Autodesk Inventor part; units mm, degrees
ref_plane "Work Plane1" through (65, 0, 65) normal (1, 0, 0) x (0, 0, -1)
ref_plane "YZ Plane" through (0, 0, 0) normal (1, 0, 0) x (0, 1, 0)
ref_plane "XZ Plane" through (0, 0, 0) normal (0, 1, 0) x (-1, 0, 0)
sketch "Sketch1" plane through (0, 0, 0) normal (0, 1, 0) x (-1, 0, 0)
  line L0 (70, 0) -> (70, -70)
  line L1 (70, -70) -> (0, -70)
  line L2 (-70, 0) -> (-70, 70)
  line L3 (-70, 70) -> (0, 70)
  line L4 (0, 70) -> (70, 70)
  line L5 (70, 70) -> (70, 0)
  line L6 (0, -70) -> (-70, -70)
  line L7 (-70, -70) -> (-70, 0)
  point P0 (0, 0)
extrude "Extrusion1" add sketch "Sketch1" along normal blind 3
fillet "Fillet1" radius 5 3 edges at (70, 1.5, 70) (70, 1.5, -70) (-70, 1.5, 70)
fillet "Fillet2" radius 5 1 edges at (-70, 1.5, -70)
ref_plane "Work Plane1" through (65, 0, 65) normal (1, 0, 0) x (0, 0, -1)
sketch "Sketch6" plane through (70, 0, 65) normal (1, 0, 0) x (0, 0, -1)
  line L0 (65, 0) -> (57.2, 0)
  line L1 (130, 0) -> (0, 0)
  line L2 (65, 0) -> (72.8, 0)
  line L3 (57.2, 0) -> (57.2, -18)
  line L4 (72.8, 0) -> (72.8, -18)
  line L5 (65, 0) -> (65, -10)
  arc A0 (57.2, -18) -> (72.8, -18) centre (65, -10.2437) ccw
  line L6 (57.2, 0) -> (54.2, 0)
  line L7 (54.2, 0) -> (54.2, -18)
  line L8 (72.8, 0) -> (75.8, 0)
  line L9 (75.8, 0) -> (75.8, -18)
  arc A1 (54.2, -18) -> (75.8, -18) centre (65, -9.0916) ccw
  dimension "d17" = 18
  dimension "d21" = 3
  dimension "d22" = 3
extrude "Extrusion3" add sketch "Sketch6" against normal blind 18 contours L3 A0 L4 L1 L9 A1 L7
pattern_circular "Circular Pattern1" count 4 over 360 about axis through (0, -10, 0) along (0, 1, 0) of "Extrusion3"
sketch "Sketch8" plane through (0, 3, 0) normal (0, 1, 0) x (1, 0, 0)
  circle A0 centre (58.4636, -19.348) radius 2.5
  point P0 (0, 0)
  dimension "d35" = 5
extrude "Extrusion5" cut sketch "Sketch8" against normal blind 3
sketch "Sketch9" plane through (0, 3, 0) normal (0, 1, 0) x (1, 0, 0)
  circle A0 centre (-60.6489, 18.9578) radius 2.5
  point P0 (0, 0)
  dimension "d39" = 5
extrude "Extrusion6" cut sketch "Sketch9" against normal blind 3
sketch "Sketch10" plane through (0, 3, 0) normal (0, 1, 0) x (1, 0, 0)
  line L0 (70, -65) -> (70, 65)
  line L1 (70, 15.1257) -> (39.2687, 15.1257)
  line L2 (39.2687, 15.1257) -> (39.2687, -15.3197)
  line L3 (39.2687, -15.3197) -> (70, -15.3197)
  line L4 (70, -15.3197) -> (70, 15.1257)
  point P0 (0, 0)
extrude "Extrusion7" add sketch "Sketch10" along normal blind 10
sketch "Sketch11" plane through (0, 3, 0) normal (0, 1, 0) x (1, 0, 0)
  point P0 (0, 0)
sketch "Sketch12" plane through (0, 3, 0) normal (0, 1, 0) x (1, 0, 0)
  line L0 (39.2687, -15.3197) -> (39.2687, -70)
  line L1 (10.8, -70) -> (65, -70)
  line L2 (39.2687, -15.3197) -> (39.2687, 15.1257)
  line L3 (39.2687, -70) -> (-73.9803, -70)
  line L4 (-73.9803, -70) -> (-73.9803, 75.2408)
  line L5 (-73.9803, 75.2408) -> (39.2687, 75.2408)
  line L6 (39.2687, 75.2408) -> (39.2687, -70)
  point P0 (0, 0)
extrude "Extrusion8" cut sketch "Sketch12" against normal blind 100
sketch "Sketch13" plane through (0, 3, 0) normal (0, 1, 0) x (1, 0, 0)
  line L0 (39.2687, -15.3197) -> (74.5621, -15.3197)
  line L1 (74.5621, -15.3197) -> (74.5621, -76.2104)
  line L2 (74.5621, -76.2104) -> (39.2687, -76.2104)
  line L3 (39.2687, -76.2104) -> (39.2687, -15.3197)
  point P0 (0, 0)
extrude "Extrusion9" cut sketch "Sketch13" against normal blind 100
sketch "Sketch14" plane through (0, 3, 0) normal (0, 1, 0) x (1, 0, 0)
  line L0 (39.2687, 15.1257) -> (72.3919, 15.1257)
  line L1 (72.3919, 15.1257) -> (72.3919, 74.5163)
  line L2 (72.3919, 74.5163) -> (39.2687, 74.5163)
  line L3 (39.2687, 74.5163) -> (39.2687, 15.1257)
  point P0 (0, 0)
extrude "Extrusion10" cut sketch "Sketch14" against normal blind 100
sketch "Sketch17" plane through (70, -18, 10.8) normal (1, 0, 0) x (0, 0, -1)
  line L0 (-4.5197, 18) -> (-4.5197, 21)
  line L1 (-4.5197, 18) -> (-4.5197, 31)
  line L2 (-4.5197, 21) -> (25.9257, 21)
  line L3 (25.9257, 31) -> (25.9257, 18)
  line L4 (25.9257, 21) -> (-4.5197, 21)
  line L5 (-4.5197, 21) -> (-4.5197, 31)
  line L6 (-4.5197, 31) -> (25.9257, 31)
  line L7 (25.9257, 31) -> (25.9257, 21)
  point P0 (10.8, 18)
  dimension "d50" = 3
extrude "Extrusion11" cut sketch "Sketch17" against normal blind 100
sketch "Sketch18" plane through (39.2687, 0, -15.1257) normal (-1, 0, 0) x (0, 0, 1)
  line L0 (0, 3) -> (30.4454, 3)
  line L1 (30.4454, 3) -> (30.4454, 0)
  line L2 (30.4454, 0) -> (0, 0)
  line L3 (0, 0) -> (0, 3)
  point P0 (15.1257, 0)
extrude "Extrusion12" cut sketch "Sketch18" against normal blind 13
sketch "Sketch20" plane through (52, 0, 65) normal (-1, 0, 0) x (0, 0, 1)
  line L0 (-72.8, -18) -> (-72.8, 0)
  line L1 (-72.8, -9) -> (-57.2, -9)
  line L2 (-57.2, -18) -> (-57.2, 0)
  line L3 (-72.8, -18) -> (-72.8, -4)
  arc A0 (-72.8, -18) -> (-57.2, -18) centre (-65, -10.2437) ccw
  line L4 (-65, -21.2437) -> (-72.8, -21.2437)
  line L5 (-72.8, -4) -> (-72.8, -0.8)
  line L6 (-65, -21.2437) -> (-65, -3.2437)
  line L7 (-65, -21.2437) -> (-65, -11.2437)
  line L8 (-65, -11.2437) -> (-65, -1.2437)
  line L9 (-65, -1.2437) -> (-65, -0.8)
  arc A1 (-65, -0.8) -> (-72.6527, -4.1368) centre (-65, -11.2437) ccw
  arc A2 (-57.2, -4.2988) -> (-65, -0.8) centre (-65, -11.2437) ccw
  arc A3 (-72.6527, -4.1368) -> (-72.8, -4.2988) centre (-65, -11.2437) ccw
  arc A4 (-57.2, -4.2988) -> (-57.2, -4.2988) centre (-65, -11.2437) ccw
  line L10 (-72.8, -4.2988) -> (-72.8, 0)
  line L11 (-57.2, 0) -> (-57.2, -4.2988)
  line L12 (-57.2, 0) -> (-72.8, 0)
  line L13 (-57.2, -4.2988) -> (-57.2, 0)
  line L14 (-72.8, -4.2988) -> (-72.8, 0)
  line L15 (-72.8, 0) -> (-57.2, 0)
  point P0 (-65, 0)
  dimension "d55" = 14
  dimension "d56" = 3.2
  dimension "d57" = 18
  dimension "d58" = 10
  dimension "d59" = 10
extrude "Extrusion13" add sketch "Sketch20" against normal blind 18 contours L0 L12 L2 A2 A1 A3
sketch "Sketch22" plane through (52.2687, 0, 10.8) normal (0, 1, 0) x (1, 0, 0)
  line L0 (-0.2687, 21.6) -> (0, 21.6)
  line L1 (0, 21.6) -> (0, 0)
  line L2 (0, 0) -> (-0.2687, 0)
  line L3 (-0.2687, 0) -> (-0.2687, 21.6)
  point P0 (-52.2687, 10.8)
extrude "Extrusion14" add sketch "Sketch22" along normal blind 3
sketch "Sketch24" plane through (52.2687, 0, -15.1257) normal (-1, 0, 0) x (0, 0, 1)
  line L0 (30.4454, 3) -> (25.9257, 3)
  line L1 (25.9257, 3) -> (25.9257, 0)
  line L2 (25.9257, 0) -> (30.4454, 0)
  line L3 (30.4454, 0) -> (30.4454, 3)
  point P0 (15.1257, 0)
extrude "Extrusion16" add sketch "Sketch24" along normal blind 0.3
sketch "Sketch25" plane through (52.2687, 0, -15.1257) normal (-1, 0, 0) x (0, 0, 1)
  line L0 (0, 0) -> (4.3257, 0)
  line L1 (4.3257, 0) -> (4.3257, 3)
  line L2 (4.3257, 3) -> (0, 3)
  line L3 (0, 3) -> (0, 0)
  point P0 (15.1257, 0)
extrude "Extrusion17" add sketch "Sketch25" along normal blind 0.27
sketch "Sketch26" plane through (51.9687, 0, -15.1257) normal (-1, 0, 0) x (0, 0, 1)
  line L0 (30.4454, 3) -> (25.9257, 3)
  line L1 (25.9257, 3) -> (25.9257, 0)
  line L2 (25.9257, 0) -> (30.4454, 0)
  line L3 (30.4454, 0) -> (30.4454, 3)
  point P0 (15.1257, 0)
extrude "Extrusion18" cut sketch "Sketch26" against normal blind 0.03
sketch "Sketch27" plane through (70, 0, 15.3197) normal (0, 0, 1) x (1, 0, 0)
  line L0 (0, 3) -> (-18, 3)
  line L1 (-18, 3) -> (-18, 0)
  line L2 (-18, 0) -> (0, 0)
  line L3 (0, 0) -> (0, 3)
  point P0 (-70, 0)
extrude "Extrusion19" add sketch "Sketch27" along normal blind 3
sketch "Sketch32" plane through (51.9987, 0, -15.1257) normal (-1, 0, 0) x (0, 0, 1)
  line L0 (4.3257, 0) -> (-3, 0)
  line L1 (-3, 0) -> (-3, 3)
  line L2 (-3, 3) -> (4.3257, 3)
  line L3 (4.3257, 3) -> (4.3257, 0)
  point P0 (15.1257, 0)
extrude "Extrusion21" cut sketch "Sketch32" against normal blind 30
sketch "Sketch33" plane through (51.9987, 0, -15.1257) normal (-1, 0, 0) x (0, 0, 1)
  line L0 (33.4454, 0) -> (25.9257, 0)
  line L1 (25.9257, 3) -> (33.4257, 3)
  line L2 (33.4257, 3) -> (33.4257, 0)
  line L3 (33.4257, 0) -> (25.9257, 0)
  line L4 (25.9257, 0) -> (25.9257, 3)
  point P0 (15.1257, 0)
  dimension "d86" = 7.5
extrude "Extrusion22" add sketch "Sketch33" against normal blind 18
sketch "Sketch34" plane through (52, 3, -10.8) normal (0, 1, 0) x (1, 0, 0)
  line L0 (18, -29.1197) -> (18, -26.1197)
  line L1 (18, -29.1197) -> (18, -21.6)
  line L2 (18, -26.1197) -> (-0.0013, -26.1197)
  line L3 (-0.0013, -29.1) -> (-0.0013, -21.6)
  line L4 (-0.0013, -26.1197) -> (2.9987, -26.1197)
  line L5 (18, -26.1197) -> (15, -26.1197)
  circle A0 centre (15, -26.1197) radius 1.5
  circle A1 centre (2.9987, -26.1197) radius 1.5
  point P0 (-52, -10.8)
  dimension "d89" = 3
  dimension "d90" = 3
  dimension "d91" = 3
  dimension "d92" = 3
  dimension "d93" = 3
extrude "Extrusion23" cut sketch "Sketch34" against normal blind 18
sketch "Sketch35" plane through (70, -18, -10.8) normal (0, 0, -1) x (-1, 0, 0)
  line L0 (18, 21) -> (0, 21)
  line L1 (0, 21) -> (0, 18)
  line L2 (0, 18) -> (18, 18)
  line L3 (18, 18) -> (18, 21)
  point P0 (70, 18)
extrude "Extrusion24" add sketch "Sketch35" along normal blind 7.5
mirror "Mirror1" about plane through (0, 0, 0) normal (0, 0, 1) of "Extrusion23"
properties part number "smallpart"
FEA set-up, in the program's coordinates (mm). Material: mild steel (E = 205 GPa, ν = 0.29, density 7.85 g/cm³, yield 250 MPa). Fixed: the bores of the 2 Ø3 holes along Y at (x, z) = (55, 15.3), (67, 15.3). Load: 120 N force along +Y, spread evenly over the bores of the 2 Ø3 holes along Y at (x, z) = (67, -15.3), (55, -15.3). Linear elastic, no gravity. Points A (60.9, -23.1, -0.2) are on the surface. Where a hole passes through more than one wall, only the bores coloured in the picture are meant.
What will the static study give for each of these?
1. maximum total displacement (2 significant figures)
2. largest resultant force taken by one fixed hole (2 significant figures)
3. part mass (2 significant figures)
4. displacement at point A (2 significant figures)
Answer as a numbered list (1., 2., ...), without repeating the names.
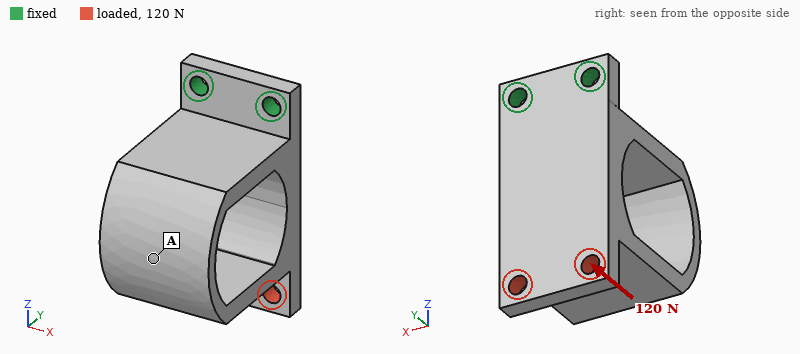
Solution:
1. 81 µm
2. 60 N
3. 40 g
4. 69 µm
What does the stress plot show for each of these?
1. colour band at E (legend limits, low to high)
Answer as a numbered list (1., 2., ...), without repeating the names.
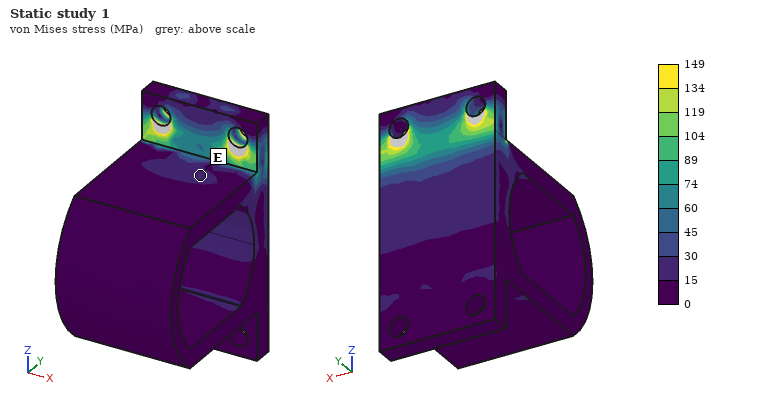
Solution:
1. 15 to 30 MPa
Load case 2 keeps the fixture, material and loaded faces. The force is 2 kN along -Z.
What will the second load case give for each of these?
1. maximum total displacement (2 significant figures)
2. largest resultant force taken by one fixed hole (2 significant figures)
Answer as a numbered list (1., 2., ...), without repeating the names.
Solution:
1. 16 µm
2. 1.0 kN
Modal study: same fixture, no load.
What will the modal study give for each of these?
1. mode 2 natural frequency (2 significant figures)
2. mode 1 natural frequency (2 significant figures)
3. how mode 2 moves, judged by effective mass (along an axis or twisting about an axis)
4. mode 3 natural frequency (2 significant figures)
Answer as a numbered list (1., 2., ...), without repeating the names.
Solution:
1. 5100 Hz
2. 1600 Hz
3. along X
4. 8300 Hz
